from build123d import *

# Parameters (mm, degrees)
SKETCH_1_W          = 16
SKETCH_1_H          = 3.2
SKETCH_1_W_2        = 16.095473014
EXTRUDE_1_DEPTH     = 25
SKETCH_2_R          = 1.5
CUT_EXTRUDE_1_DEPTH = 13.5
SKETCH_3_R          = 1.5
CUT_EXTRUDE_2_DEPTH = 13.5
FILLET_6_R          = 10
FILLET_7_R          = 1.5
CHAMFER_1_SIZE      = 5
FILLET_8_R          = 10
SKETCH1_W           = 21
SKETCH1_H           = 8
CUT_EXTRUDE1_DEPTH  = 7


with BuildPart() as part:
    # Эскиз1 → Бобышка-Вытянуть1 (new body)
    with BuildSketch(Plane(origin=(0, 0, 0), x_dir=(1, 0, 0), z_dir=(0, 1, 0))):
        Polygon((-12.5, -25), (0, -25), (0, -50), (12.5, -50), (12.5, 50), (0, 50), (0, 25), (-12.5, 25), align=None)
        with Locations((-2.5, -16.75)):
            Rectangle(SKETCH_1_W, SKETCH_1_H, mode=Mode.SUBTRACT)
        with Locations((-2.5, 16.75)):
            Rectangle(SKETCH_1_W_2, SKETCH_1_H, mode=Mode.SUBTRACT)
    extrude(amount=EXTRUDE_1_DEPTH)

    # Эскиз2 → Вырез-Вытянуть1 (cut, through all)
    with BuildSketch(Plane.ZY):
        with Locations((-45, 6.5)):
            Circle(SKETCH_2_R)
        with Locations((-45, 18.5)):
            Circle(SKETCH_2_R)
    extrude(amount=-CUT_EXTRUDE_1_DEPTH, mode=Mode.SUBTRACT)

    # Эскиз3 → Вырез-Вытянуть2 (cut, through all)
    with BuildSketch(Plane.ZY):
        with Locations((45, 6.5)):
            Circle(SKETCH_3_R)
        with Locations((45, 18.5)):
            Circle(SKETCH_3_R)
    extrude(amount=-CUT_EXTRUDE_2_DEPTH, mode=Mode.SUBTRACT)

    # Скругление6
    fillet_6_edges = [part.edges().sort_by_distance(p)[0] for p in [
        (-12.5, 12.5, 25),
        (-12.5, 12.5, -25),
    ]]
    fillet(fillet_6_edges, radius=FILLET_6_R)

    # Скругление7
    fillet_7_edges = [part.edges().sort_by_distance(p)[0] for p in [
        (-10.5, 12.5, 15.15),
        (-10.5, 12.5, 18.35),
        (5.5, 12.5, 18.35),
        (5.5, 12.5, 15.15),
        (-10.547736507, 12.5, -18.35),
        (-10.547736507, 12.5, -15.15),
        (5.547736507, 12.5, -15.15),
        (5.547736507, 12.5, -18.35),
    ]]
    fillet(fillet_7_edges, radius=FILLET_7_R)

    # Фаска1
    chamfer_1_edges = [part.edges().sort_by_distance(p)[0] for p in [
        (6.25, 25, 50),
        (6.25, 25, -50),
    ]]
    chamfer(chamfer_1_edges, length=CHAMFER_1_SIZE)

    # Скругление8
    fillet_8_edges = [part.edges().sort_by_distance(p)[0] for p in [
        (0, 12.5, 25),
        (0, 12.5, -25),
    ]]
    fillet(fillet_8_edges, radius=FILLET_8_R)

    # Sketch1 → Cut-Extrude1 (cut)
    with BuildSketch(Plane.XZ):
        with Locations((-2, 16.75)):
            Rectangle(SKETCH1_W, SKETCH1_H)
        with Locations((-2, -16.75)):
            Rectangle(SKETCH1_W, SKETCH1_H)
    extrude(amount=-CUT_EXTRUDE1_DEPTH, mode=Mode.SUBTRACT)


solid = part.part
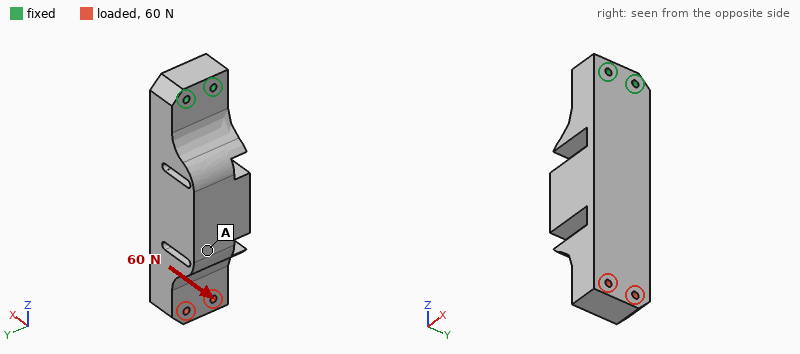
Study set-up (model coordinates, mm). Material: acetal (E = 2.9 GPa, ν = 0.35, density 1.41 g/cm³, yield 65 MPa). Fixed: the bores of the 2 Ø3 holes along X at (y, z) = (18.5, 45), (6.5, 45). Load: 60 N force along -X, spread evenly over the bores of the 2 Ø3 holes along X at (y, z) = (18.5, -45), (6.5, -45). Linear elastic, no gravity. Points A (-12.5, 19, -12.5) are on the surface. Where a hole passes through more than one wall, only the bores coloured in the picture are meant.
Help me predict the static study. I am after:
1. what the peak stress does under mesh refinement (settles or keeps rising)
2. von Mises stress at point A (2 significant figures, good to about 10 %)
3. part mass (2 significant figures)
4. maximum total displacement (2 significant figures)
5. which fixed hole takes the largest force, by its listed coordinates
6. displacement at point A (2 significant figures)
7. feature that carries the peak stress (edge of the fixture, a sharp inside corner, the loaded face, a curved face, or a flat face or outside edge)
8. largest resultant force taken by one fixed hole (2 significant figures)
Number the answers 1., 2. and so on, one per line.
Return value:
1. keeps rising
2. 2.4 MPa
3. 59 g
4. 1.1 mm
5. (6.5, 45)
6. 0.59 mm
7. edge of the fixture
8. 34 N
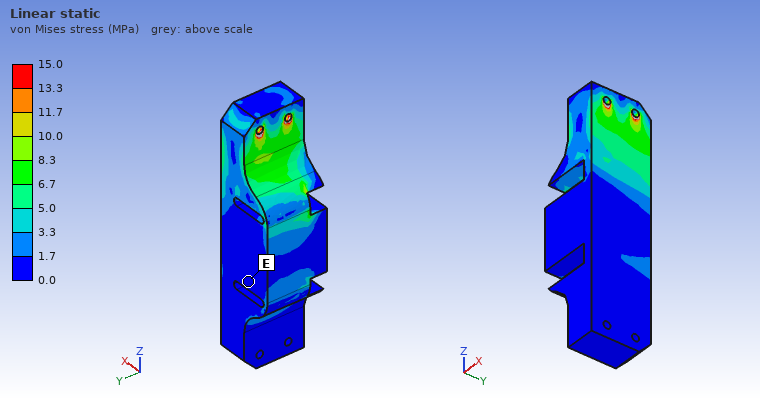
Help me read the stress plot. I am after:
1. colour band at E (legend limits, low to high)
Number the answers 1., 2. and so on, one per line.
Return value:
1. 0.0 to 1.7 MPa
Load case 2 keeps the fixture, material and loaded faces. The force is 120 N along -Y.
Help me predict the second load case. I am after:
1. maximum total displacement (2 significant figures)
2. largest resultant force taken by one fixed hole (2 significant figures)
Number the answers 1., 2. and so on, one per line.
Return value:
1. 1.0 mm
2. 770 N
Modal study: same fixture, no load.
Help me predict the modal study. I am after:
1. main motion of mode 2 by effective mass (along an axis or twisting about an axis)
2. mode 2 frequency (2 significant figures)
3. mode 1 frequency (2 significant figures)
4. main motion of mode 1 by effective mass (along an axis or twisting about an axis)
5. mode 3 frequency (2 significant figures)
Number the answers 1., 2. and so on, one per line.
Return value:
1. along Y
2. 470 Hz
3. 310 Hz
4. along X
5. 1500 Hz
